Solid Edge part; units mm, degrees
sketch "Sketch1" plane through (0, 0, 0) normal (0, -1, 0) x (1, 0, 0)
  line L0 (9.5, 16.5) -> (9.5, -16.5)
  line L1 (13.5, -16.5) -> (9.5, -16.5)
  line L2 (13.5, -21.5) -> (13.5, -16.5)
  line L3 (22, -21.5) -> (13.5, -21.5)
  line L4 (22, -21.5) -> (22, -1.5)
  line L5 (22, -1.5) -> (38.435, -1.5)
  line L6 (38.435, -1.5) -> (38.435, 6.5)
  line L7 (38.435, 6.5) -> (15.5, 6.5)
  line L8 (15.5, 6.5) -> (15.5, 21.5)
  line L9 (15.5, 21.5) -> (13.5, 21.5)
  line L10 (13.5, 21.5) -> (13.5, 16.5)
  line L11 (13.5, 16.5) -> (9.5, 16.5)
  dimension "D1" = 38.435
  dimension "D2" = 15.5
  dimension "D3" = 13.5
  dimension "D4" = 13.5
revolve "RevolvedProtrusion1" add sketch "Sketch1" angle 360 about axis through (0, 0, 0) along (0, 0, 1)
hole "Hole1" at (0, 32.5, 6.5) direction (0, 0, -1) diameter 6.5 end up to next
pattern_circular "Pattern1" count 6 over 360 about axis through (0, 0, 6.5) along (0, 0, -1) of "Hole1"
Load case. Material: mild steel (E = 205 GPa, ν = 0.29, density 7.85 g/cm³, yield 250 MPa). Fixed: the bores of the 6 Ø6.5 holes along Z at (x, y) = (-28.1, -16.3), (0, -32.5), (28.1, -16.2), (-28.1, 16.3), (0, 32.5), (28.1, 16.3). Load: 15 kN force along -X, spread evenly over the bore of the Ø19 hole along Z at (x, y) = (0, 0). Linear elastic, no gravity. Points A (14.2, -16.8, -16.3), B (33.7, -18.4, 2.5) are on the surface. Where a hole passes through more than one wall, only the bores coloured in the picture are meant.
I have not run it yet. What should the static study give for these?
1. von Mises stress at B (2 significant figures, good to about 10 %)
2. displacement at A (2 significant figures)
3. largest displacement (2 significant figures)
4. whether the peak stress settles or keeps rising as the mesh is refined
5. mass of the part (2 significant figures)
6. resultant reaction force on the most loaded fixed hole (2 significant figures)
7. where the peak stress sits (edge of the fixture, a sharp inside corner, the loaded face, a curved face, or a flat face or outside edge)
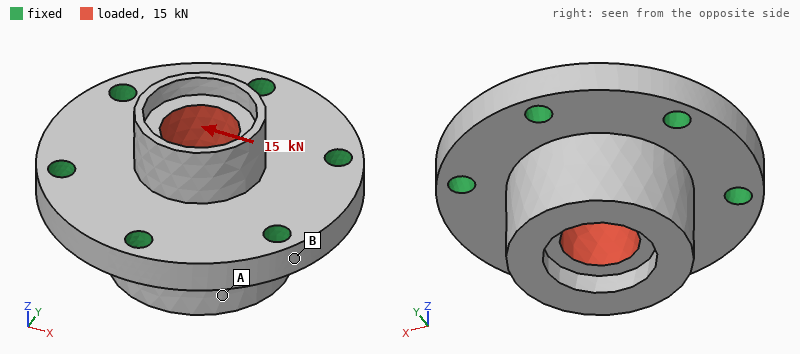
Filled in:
10.0 MPa
2.7 µm
3.9 µm
keeps rising
490 g
3.2 kN
edge of the fixture
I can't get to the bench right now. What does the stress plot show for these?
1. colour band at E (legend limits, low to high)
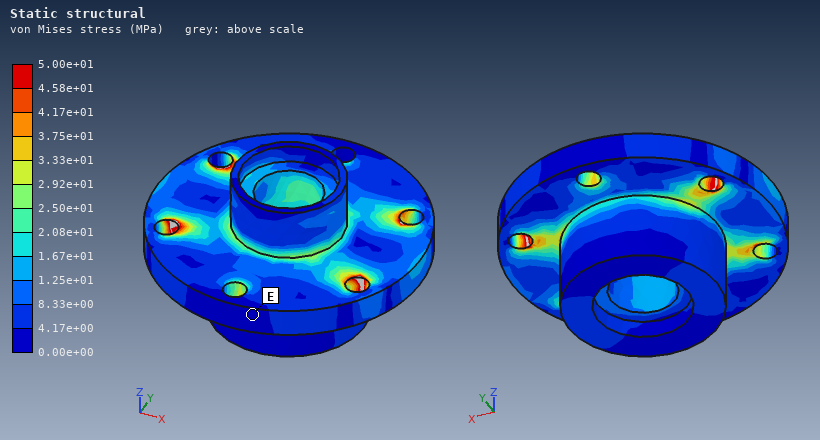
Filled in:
0.00e+00 to 4.17e+00 MPa
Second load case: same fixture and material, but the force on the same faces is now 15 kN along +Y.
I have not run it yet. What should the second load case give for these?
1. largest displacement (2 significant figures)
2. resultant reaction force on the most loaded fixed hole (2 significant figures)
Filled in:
3.9 µm
3.6 kN
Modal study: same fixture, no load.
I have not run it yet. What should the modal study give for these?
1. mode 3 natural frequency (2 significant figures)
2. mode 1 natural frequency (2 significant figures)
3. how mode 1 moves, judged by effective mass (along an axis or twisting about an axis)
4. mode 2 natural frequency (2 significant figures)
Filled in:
16 kHz
14 kHz
along Z
16 kHz
